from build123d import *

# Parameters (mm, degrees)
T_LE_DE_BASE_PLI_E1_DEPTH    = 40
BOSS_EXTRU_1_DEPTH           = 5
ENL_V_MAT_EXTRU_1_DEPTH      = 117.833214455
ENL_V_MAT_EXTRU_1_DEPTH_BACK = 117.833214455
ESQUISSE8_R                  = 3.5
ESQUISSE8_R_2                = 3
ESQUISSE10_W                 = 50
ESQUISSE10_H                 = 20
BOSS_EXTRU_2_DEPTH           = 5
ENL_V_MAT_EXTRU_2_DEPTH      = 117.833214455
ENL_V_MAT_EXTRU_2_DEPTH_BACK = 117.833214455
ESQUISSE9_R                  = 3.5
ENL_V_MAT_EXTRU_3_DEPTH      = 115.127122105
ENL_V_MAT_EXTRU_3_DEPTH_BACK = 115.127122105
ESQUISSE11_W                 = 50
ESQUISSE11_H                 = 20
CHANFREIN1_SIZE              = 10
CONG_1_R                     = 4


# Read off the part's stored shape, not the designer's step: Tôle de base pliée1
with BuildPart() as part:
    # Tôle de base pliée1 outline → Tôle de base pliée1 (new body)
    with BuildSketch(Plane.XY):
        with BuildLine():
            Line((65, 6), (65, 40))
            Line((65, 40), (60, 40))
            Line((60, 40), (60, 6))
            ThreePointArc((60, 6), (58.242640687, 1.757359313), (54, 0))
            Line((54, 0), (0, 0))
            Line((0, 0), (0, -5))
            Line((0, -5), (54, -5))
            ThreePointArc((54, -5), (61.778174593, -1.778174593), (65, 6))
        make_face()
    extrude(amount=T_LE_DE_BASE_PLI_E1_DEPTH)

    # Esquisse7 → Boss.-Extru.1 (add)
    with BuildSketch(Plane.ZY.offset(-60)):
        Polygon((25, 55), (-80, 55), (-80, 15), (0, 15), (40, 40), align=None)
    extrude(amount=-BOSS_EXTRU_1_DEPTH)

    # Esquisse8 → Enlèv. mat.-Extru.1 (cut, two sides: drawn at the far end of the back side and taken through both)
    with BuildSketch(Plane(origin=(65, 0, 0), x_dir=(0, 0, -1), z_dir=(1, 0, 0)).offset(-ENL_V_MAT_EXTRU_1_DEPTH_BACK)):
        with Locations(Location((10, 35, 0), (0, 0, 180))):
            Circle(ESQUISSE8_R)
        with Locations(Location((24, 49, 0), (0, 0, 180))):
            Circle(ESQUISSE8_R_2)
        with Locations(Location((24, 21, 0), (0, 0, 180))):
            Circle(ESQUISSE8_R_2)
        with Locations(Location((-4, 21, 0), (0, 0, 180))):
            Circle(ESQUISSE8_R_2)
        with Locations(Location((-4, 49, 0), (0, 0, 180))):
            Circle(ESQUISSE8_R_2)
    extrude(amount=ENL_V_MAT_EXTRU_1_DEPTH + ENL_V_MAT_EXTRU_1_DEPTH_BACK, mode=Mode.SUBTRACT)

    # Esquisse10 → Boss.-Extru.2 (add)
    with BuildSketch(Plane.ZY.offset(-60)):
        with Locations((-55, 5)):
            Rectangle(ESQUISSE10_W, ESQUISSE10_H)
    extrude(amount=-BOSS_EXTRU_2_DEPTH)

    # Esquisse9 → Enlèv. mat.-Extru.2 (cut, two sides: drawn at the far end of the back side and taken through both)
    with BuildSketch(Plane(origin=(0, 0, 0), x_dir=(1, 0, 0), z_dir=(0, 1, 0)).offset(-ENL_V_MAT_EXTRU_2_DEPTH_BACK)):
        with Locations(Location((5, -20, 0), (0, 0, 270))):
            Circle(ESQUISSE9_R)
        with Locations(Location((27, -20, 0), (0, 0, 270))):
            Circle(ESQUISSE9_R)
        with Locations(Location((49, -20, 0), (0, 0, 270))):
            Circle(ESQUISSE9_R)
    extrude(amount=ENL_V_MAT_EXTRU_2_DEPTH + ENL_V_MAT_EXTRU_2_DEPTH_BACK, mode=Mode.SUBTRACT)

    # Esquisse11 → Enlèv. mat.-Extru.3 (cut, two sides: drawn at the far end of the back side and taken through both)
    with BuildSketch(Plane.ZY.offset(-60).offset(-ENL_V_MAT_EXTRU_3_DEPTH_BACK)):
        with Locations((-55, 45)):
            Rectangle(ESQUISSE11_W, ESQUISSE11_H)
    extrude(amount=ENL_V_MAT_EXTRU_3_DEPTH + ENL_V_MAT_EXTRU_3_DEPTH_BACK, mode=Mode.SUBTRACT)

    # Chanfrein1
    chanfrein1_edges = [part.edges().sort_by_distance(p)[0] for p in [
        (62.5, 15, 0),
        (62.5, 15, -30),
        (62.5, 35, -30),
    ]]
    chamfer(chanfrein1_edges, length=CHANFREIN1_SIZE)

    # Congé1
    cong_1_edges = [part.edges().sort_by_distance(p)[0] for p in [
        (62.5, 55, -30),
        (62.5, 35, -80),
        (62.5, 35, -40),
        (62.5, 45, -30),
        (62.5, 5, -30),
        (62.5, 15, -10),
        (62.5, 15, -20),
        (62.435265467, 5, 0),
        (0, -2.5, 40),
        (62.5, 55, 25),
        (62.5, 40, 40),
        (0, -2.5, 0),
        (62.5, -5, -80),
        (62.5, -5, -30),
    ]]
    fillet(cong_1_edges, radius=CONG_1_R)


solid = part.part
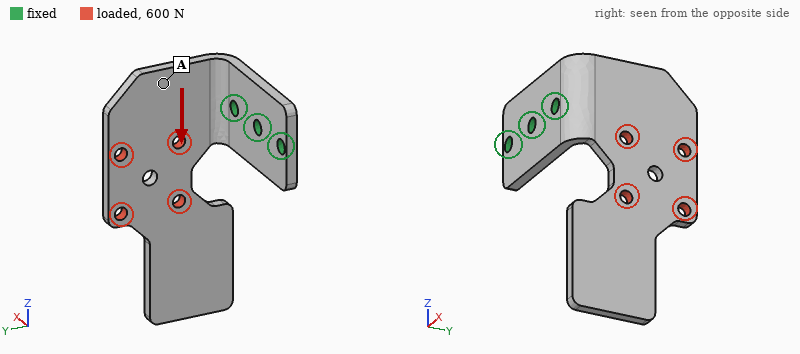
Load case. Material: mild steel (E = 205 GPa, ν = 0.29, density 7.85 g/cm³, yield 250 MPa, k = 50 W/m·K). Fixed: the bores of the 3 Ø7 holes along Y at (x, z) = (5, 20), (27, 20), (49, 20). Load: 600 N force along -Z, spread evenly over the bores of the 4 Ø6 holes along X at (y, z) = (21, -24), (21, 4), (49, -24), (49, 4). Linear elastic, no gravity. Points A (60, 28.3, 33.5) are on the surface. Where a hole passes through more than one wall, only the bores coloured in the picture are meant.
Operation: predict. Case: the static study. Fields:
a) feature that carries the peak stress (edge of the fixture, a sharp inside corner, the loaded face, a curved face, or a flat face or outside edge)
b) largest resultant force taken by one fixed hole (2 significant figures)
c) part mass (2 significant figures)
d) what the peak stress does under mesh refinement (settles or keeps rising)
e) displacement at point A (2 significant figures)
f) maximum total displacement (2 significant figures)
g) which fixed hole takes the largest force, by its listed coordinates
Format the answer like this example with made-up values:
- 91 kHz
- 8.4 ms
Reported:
- edge of the fixture
- 730 N
- 300 g
- keeps rising
- 0.060 mm
- 0.20 mm
- (49, 20)
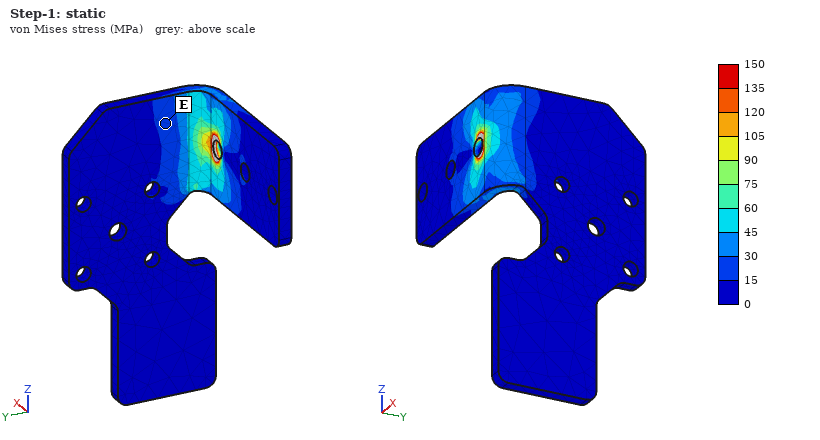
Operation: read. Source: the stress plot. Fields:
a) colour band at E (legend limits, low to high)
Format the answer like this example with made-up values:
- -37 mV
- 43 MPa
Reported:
- 15 to 30 MPa
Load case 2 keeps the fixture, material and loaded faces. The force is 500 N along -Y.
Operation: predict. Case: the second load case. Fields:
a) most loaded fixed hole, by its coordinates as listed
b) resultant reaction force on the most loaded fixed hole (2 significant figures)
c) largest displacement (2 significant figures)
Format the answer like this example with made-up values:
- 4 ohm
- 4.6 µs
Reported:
- (49, 20)
- 580 N
- 0.16 mm
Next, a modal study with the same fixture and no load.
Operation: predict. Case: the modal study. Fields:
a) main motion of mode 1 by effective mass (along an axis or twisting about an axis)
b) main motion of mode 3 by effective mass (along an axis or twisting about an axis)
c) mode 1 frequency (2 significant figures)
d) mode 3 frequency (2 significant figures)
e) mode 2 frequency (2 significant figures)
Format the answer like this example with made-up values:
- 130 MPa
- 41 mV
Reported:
- along X
- along X
- 360 Hz
- 780 Hz
- 670 Hz
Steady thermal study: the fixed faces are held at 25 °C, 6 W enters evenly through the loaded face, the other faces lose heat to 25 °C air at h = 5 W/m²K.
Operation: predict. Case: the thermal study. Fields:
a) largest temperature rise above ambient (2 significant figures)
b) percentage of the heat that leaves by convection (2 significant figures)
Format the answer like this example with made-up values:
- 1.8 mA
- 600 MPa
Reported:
- 31 K
- 23 %
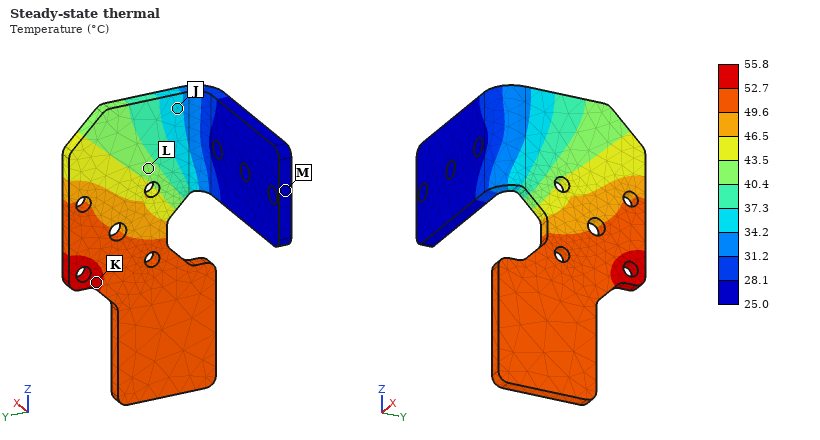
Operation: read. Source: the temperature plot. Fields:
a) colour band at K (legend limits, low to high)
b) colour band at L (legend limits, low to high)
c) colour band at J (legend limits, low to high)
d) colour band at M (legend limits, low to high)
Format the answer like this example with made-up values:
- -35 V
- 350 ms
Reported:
- 52.7 to 55.8 °C
- 40.4 to 43.5 °C
- 34.2 to 37.3 °C
- 25.0 to 28.1 °C
